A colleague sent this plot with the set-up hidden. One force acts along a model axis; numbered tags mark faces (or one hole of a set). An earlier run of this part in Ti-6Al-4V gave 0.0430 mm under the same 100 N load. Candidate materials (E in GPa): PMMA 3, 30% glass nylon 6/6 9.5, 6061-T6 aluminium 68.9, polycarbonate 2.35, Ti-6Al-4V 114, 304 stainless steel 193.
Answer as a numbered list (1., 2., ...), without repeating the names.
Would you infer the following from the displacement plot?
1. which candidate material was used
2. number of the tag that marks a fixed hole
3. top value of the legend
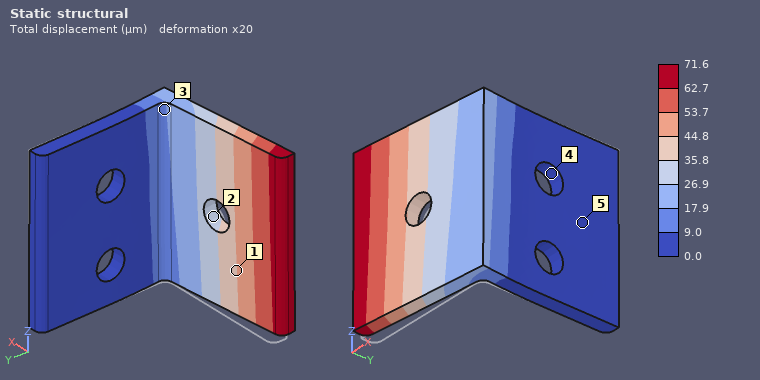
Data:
1. 6061-T6 aluminium
2. 4
3. 71.6 µm
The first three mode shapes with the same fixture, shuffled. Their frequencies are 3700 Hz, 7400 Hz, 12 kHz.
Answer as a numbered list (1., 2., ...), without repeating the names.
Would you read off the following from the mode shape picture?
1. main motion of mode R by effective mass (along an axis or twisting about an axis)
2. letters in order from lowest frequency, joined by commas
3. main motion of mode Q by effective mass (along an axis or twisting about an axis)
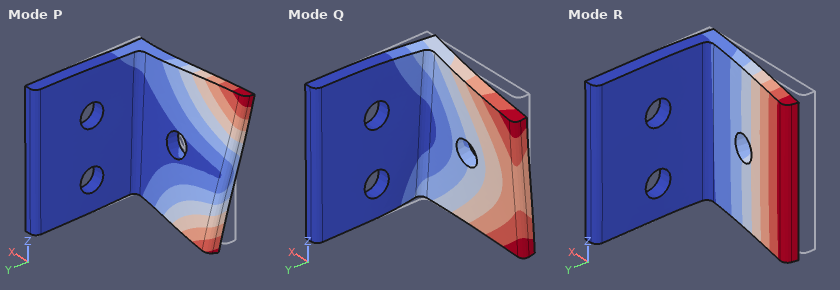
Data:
1. along Y
2. R, Q, P
3. along Z
